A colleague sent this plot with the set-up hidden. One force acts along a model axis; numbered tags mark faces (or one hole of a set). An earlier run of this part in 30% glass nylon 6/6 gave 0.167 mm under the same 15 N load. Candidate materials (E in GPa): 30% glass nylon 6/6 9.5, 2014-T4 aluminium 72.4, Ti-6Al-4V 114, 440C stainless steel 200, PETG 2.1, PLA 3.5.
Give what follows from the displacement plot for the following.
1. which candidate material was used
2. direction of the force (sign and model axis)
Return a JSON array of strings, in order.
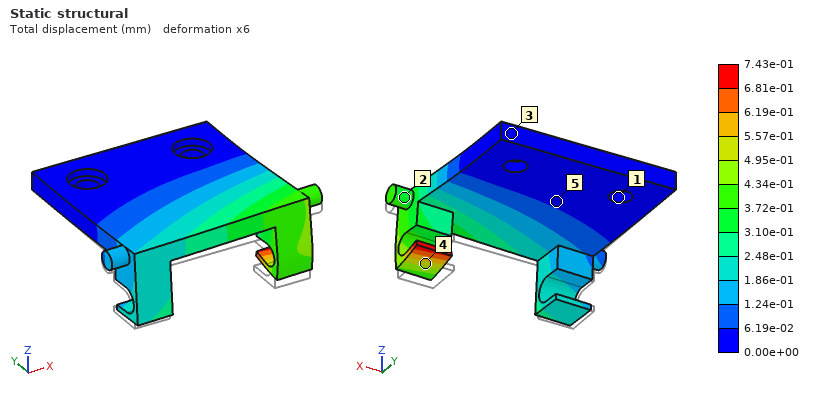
["PETG", "+Z"]
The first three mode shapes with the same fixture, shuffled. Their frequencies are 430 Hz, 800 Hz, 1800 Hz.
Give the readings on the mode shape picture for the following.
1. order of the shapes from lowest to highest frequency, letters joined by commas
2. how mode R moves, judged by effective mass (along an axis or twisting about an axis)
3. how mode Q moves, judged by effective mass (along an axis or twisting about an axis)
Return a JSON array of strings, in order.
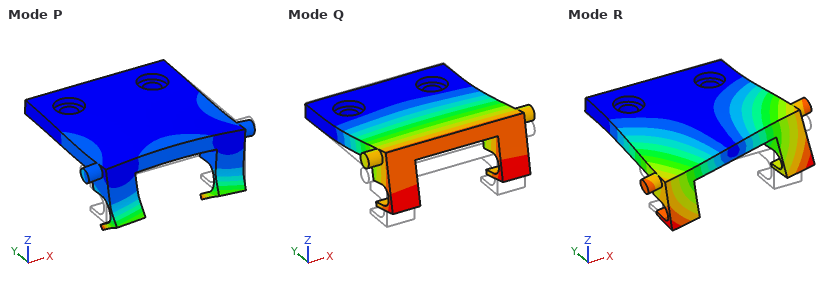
["Q, R, P", "twisting about Y", "along Z"]
